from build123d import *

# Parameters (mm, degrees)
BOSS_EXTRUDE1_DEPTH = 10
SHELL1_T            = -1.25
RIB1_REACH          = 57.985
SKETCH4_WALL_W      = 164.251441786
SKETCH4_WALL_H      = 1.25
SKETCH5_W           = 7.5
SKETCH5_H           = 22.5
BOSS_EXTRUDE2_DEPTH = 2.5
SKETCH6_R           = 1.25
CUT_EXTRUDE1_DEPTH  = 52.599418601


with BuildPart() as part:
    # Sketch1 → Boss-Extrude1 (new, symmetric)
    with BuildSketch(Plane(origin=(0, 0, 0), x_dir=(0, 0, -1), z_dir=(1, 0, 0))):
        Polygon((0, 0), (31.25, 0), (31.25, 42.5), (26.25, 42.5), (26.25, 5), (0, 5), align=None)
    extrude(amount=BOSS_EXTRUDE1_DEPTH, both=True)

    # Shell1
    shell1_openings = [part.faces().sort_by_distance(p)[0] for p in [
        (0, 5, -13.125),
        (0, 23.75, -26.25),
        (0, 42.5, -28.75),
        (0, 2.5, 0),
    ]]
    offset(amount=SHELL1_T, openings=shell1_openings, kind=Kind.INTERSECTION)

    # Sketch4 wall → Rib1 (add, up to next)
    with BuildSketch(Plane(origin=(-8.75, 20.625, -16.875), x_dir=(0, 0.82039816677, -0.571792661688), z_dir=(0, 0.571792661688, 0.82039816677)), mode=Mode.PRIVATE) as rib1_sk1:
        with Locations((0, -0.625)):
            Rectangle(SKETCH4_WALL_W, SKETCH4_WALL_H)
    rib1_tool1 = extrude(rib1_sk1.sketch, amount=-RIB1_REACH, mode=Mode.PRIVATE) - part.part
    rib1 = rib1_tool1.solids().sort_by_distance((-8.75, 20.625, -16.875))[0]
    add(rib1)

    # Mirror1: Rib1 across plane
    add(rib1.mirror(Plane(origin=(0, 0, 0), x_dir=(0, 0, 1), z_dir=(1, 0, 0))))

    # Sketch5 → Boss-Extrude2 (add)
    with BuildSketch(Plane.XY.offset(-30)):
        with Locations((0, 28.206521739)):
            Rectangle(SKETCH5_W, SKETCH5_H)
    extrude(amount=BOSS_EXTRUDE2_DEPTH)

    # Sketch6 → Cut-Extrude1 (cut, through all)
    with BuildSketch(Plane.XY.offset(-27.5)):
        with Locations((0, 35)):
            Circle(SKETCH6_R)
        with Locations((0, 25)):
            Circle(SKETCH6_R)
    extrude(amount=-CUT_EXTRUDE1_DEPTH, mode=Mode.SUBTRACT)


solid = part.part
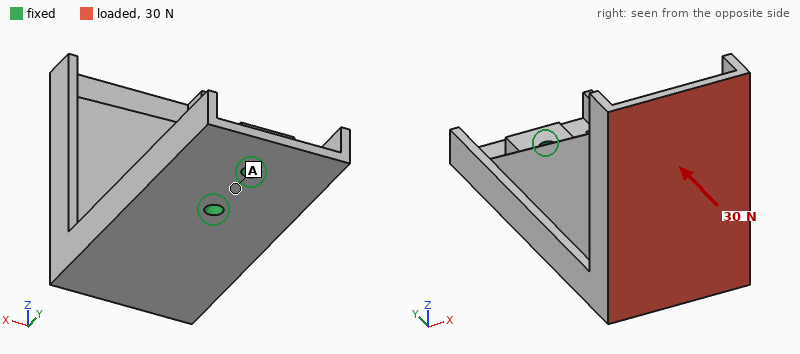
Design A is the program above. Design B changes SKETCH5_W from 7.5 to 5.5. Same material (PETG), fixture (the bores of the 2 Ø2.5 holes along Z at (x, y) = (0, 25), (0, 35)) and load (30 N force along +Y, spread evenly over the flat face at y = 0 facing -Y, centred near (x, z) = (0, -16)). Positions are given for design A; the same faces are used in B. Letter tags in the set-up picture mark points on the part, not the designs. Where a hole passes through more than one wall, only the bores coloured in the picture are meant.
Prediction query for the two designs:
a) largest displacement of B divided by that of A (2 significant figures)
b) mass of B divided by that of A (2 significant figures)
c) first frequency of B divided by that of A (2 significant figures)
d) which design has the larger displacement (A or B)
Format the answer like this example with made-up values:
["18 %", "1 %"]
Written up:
["1.2", "0.97", "0.91", "B"]
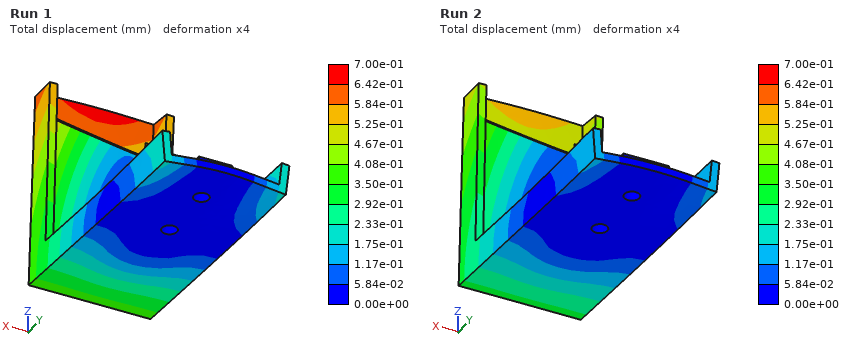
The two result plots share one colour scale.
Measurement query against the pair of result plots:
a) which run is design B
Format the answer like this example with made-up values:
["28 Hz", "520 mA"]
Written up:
["Run 1"]
